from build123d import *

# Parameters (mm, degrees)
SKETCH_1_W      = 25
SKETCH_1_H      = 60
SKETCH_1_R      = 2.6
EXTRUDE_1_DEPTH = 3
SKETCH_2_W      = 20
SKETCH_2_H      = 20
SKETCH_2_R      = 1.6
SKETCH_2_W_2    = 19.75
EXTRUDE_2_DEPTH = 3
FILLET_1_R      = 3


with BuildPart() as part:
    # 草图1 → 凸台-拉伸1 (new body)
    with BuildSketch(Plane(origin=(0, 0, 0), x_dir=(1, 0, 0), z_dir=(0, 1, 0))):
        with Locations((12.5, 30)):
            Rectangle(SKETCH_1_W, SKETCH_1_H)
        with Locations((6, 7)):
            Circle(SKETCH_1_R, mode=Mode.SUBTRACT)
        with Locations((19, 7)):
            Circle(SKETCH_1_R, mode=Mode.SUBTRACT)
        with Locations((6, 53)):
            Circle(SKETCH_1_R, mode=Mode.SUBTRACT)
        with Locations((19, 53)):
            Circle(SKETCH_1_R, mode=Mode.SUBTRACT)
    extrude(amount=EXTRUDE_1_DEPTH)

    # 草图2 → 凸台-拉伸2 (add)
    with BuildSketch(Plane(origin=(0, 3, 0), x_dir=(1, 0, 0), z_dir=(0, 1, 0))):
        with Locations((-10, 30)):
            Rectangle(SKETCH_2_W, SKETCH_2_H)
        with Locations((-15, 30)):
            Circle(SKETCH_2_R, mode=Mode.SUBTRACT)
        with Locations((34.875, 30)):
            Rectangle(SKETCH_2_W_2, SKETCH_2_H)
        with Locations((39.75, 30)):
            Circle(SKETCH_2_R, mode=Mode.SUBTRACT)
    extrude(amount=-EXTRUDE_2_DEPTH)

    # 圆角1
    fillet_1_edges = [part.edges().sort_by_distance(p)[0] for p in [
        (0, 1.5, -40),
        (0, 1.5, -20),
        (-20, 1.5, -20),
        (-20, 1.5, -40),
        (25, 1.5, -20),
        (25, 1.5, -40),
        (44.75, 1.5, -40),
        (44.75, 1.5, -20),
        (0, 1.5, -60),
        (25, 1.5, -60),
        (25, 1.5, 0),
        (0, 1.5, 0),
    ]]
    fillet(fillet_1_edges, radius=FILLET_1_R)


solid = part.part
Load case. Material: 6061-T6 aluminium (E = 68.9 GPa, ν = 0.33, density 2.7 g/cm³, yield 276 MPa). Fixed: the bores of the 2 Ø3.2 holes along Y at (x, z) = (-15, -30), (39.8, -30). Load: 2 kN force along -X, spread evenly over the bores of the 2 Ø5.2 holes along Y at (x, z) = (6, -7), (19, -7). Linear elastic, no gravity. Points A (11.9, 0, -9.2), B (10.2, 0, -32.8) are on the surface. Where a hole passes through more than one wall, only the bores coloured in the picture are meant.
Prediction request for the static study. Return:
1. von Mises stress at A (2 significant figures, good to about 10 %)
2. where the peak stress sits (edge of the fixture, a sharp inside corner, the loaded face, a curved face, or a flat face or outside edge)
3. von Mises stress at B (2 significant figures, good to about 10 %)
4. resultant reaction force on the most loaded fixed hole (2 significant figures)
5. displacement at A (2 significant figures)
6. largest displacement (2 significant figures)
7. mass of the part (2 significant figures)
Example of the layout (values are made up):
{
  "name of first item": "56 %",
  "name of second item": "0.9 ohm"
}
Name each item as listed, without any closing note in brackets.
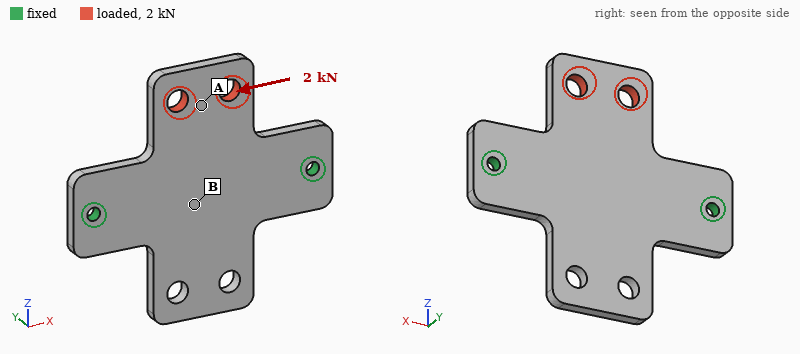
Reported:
{
  "von Mises stress at A": "56 MPa",
  "where the peak stress sits": "a curved face",
  "von Mises stress at B": "19 MPa",
  "resultant reaction force on the most loaded fixed hole": "1.3 kN",
  "displacement at A": "39 µm",
  "largest displacement": "64 µm",
  "mass of the part": "18 g"
}
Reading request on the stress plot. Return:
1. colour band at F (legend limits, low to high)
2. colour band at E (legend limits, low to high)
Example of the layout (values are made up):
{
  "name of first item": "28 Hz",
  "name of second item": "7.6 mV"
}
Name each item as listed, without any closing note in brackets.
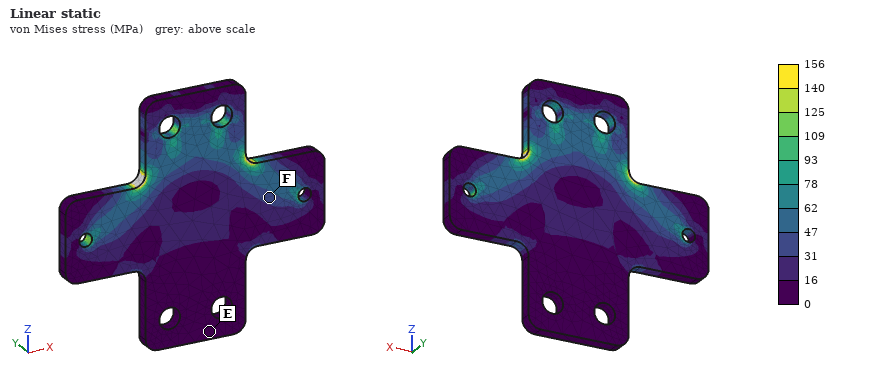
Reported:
{
  "colour band at F": "31 to 47 MPa",
  "colour band at E": "0 to 16 MPa"
}
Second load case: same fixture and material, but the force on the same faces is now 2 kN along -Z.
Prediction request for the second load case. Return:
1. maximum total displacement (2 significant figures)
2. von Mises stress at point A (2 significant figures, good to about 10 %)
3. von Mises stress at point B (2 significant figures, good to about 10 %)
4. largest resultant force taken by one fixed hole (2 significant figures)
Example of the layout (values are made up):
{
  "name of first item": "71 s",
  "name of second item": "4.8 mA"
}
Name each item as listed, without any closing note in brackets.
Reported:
{
  "maximum total displacement": "33 µm",
  "von Mises stress at point A": "20 MPa",
  "von Mises stress at point B": "17 MPa",
  "largest resultant force taken by one fixed hole": "1.0 kN"
}
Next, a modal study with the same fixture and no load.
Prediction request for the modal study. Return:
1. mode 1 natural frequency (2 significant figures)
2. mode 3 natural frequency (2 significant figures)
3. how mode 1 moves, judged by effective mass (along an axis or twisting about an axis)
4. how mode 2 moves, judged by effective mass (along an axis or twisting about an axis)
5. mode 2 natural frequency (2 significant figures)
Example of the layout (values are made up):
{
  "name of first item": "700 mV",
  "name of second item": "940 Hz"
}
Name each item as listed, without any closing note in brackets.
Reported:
{
  "mode 1 natural frequency": "1900 Hz",
  "mode 3 natural frequency": "6700 Hz",
  "how mode 1 moves, judged by effective mass": "twisting about X",
  "how mode 2 moves, judged by effective mass": "along Y",
  "mode 2 natural frequency": "2600 Hz"
}
